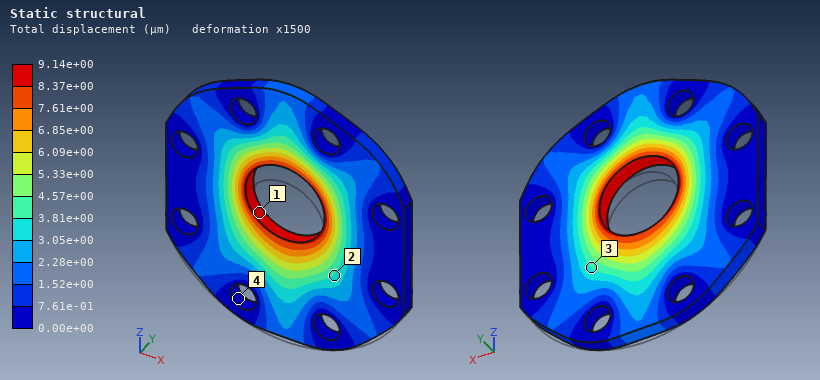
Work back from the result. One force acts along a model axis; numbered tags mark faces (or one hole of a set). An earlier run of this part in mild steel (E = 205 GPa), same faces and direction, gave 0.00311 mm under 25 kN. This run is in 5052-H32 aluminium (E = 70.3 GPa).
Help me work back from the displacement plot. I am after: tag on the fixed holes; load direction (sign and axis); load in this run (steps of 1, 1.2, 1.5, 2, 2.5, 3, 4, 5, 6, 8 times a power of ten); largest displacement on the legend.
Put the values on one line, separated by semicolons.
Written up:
4; +Z; 25 kN; 9.14e+00 µm
